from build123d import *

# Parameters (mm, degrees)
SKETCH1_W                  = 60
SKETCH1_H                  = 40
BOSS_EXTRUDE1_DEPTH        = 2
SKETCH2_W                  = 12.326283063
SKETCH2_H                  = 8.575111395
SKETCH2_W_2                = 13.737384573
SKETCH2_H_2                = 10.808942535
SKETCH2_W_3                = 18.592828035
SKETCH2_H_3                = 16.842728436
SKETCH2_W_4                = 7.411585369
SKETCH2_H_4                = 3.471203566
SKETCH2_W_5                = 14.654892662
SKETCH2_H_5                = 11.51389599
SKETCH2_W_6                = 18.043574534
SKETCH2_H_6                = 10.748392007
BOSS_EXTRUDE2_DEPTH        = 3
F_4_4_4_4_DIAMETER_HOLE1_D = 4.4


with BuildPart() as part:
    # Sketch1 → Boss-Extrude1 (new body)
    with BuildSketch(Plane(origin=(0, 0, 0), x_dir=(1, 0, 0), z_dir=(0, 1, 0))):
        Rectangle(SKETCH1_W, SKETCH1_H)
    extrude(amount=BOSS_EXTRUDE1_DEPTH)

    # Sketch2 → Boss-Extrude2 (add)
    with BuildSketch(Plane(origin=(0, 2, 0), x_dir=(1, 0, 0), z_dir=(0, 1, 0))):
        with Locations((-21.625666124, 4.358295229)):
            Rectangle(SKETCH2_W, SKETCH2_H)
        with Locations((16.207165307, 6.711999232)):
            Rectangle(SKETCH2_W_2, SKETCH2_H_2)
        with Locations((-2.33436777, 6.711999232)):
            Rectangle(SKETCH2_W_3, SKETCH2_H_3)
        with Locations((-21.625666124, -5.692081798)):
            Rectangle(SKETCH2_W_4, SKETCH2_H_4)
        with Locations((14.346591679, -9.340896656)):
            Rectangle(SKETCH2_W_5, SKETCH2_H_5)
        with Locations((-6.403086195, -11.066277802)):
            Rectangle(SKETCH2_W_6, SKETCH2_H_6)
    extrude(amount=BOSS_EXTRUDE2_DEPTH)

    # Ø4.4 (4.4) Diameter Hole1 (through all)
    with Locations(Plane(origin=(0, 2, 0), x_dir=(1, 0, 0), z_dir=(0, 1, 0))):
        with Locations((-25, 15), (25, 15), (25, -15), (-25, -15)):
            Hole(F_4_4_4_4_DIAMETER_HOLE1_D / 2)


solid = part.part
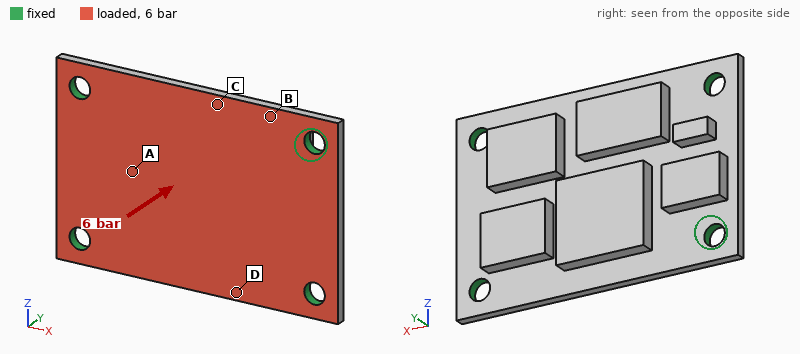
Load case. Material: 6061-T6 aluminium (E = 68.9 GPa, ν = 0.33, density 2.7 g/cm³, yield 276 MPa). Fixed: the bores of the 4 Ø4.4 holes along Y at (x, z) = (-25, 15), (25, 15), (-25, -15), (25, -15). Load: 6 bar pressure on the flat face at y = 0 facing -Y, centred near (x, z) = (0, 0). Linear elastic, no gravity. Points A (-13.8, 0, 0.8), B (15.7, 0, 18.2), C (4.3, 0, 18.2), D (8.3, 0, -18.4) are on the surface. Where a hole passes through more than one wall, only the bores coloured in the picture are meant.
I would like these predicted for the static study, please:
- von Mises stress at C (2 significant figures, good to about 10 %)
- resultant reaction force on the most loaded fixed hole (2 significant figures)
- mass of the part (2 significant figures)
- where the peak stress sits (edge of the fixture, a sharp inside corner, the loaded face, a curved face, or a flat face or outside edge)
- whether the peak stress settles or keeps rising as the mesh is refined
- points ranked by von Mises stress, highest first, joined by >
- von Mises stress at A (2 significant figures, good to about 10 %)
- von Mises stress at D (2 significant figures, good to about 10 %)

81 MPa
410 N
20 g
edge of the fixture
keeps rising
C > D > A > B
44 MPa
67 MPa
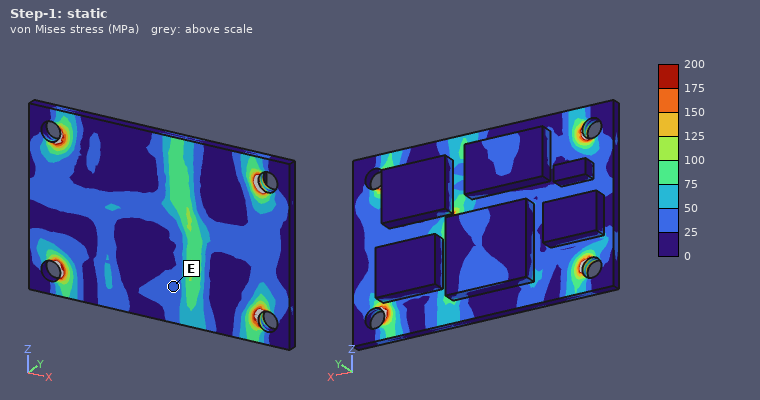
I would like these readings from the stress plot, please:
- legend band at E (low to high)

25 to 50 MPa
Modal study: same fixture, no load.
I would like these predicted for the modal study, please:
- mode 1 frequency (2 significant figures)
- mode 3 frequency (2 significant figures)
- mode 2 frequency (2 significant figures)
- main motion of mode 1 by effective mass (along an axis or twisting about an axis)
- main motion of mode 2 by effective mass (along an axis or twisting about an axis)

4200 Hz
11 kHz
7200 Hz
along Y
twisting about X
